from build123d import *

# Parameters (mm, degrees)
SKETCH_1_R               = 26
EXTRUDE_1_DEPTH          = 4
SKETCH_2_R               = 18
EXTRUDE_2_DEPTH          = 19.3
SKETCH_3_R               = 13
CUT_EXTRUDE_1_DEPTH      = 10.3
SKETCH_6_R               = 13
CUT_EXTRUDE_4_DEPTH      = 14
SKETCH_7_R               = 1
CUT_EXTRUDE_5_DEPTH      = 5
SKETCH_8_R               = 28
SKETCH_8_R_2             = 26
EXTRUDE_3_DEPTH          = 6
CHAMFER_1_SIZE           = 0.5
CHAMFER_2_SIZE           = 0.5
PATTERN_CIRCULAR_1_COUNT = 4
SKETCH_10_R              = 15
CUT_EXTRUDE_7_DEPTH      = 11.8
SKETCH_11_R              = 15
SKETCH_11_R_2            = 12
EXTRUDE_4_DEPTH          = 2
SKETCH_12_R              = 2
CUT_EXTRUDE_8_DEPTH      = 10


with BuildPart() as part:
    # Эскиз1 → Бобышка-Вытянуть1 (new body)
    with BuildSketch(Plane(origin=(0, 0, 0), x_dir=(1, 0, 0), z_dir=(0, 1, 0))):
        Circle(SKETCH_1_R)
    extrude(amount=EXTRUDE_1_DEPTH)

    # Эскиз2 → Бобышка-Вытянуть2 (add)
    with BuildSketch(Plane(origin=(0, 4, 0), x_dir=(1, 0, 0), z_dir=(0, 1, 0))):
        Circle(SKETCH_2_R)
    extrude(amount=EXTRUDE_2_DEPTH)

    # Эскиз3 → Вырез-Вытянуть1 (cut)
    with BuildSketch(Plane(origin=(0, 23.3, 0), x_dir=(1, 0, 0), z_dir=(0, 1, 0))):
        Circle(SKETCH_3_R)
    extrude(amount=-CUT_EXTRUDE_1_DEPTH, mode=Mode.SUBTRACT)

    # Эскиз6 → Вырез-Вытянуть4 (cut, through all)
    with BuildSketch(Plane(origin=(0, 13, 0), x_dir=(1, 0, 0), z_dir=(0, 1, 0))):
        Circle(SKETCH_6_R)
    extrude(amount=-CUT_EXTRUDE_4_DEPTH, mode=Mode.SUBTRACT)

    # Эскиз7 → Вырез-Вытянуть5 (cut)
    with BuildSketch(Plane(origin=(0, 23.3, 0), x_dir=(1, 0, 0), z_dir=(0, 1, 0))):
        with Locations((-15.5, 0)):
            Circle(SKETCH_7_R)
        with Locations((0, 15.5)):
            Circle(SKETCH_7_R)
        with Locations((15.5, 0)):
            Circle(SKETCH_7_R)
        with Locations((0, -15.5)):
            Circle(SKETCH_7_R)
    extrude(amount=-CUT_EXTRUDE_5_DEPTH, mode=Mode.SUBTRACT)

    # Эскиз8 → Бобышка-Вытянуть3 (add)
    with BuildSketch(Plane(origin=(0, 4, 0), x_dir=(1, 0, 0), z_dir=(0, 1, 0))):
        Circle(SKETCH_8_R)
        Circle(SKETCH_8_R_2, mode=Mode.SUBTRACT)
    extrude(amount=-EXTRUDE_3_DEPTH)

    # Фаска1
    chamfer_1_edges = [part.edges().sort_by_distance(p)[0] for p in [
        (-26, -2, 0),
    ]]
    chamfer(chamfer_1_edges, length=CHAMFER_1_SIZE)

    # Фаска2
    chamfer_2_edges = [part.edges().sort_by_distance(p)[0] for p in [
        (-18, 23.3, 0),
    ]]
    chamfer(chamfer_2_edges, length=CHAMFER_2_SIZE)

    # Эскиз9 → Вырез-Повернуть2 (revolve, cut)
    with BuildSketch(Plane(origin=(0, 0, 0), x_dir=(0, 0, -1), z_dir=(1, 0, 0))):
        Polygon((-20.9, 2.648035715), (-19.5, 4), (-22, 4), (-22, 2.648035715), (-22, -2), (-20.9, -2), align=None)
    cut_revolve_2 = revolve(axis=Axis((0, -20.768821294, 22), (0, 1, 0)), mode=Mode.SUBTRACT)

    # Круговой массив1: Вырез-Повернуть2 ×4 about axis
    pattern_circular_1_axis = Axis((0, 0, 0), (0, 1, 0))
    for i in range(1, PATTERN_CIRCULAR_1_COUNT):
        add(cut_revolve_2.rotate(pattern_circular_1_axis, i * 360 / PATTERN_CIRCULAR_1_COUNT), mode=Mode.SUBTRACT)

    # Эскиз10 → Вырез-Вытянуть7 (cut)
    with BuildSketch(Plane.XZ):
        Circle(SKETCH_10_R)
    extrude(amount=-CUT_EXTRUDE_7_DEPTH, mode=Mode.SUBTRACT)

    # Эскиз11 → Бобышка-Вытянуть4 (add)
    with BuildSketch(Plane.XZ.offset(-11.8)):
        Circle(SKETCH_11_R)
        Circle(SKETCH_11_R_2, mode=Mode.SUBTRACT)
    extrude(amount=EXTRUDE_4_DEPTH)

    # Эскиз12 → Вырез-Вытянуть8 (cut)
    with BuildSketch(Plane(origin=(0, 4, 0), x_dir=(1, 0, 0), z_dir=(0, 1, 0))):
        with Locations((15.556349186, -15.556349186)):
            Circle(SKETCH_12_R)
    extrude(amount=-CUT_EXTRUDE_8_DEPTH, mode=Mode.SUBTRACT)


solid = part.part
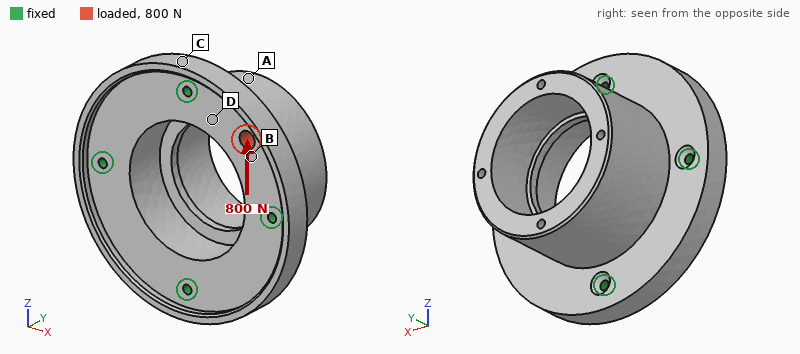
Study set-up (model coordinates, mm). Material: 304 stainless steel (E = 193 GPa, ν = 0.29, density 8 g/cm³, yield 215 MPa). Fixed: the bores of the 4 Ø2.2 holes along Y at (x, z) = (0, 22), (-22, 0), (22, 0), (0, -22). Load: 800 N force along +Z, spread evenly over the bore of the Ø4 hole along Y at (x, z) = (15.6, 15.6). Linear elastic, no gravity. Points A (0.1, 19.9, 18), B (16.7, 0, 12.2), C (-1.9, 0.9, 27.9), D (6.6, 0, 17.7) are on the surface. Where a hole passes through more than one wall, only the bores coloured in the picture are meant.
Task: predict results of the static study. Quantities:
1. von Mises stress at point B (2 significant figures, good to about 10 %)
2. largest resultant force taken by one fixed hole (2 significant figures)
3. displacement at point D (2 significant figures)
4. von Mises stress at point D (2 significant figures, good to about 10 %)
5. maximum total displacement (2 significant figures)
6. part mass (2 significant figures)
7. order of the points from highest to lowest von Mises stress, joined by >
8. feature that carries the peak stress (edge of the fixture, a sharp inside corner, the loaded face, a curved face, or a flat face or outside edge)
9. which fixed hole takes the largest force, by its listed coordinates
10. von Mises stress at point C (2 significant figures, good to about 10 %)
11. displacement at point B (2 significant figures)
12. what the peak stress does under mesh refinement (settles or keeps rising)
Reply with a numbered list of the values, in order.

1. 20 MPa
2. 580 N
3. 1.0 µm
4. 10 MPa
5. 2.1 µm
6. 130 g
7. B > D > C > A
8. edge of the fixture
9. (22, 0)
10. 5.6 MPa
11. 1.6 µm
12. keeps rising
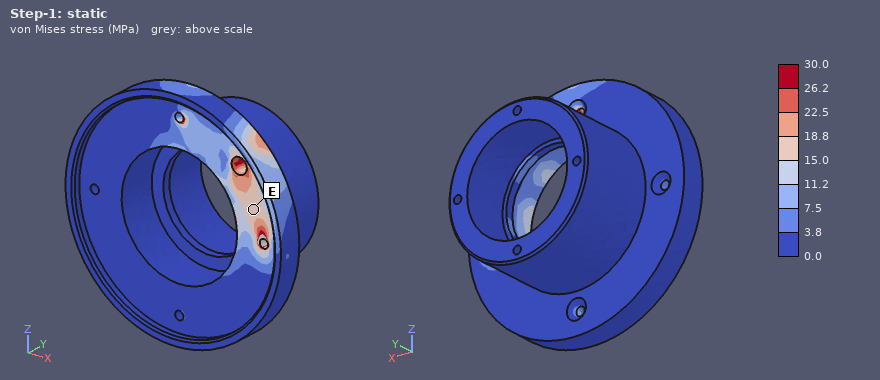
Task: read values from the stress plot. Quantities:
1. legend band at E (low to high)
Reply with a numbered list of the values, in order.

1. 15.0 to 18.8 MPa
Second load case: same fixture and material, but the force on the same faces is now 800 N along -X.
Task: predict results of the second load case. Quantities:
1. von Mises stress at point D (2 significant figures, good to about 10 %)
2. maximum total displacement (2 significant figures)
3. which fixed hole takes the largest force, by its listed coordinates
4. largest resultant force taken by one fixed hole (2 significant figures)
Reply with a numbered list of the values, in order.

1. 16 MPa
2. 2.1 µm
3. (0, 22)
4. 580 N
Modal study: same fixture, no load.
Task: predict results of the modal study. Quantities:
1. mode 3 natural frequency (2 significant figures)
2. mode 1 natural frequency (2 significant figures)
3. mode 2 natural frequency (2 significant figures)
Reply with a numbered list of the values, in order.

1. 12 kHz
2. 11 kHz
3. 11 kHz
